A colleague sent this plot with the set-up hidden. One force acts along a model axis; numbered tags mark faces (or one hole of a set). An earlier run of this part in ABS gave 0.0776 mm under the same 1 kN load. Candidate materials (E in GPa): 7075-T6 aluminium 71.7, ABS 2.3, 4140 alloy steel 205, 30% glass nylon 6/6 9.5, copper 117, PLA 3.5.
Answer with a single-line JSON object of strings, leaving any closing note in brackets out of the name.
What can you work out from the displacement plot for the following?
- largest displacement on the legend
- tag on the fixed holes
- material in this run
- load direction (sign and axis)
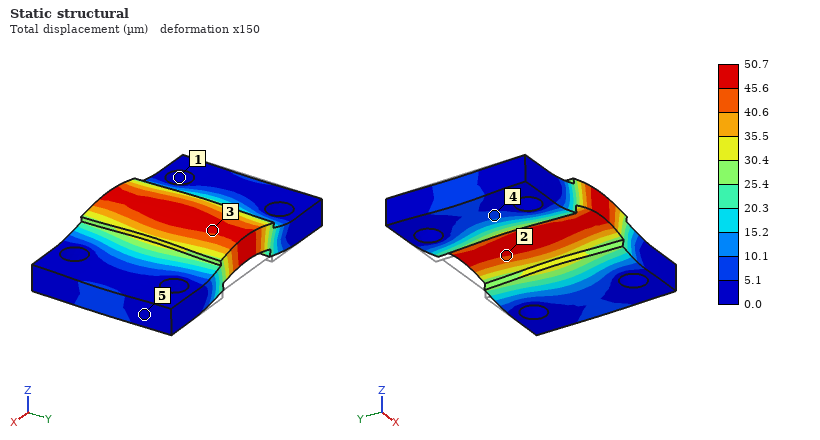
{"largest displacement on the legend": "50.7 µm", "tag on the fixed holes": "1", "material in this run": "PLA", "load direction": "+Z"}
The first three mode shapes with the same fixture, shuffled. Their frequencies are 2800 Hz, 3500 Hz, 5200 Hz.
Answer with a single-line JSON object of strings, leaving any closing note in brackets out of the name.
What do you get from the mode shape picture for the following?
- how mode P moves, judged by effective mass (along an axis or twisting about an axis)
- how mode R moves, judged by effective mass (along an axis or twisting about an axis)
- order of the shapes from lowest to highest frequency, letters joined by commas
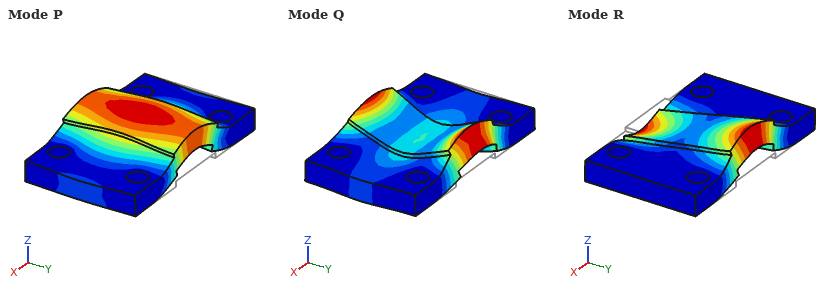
{"how mode P moves, judged by effective mass": "along Z", "how mode R moves, judged by effective mass": "twisting about X", "order of the shapes from lowest to highest frequency, letters joined by commas": "P, R, Q"}
